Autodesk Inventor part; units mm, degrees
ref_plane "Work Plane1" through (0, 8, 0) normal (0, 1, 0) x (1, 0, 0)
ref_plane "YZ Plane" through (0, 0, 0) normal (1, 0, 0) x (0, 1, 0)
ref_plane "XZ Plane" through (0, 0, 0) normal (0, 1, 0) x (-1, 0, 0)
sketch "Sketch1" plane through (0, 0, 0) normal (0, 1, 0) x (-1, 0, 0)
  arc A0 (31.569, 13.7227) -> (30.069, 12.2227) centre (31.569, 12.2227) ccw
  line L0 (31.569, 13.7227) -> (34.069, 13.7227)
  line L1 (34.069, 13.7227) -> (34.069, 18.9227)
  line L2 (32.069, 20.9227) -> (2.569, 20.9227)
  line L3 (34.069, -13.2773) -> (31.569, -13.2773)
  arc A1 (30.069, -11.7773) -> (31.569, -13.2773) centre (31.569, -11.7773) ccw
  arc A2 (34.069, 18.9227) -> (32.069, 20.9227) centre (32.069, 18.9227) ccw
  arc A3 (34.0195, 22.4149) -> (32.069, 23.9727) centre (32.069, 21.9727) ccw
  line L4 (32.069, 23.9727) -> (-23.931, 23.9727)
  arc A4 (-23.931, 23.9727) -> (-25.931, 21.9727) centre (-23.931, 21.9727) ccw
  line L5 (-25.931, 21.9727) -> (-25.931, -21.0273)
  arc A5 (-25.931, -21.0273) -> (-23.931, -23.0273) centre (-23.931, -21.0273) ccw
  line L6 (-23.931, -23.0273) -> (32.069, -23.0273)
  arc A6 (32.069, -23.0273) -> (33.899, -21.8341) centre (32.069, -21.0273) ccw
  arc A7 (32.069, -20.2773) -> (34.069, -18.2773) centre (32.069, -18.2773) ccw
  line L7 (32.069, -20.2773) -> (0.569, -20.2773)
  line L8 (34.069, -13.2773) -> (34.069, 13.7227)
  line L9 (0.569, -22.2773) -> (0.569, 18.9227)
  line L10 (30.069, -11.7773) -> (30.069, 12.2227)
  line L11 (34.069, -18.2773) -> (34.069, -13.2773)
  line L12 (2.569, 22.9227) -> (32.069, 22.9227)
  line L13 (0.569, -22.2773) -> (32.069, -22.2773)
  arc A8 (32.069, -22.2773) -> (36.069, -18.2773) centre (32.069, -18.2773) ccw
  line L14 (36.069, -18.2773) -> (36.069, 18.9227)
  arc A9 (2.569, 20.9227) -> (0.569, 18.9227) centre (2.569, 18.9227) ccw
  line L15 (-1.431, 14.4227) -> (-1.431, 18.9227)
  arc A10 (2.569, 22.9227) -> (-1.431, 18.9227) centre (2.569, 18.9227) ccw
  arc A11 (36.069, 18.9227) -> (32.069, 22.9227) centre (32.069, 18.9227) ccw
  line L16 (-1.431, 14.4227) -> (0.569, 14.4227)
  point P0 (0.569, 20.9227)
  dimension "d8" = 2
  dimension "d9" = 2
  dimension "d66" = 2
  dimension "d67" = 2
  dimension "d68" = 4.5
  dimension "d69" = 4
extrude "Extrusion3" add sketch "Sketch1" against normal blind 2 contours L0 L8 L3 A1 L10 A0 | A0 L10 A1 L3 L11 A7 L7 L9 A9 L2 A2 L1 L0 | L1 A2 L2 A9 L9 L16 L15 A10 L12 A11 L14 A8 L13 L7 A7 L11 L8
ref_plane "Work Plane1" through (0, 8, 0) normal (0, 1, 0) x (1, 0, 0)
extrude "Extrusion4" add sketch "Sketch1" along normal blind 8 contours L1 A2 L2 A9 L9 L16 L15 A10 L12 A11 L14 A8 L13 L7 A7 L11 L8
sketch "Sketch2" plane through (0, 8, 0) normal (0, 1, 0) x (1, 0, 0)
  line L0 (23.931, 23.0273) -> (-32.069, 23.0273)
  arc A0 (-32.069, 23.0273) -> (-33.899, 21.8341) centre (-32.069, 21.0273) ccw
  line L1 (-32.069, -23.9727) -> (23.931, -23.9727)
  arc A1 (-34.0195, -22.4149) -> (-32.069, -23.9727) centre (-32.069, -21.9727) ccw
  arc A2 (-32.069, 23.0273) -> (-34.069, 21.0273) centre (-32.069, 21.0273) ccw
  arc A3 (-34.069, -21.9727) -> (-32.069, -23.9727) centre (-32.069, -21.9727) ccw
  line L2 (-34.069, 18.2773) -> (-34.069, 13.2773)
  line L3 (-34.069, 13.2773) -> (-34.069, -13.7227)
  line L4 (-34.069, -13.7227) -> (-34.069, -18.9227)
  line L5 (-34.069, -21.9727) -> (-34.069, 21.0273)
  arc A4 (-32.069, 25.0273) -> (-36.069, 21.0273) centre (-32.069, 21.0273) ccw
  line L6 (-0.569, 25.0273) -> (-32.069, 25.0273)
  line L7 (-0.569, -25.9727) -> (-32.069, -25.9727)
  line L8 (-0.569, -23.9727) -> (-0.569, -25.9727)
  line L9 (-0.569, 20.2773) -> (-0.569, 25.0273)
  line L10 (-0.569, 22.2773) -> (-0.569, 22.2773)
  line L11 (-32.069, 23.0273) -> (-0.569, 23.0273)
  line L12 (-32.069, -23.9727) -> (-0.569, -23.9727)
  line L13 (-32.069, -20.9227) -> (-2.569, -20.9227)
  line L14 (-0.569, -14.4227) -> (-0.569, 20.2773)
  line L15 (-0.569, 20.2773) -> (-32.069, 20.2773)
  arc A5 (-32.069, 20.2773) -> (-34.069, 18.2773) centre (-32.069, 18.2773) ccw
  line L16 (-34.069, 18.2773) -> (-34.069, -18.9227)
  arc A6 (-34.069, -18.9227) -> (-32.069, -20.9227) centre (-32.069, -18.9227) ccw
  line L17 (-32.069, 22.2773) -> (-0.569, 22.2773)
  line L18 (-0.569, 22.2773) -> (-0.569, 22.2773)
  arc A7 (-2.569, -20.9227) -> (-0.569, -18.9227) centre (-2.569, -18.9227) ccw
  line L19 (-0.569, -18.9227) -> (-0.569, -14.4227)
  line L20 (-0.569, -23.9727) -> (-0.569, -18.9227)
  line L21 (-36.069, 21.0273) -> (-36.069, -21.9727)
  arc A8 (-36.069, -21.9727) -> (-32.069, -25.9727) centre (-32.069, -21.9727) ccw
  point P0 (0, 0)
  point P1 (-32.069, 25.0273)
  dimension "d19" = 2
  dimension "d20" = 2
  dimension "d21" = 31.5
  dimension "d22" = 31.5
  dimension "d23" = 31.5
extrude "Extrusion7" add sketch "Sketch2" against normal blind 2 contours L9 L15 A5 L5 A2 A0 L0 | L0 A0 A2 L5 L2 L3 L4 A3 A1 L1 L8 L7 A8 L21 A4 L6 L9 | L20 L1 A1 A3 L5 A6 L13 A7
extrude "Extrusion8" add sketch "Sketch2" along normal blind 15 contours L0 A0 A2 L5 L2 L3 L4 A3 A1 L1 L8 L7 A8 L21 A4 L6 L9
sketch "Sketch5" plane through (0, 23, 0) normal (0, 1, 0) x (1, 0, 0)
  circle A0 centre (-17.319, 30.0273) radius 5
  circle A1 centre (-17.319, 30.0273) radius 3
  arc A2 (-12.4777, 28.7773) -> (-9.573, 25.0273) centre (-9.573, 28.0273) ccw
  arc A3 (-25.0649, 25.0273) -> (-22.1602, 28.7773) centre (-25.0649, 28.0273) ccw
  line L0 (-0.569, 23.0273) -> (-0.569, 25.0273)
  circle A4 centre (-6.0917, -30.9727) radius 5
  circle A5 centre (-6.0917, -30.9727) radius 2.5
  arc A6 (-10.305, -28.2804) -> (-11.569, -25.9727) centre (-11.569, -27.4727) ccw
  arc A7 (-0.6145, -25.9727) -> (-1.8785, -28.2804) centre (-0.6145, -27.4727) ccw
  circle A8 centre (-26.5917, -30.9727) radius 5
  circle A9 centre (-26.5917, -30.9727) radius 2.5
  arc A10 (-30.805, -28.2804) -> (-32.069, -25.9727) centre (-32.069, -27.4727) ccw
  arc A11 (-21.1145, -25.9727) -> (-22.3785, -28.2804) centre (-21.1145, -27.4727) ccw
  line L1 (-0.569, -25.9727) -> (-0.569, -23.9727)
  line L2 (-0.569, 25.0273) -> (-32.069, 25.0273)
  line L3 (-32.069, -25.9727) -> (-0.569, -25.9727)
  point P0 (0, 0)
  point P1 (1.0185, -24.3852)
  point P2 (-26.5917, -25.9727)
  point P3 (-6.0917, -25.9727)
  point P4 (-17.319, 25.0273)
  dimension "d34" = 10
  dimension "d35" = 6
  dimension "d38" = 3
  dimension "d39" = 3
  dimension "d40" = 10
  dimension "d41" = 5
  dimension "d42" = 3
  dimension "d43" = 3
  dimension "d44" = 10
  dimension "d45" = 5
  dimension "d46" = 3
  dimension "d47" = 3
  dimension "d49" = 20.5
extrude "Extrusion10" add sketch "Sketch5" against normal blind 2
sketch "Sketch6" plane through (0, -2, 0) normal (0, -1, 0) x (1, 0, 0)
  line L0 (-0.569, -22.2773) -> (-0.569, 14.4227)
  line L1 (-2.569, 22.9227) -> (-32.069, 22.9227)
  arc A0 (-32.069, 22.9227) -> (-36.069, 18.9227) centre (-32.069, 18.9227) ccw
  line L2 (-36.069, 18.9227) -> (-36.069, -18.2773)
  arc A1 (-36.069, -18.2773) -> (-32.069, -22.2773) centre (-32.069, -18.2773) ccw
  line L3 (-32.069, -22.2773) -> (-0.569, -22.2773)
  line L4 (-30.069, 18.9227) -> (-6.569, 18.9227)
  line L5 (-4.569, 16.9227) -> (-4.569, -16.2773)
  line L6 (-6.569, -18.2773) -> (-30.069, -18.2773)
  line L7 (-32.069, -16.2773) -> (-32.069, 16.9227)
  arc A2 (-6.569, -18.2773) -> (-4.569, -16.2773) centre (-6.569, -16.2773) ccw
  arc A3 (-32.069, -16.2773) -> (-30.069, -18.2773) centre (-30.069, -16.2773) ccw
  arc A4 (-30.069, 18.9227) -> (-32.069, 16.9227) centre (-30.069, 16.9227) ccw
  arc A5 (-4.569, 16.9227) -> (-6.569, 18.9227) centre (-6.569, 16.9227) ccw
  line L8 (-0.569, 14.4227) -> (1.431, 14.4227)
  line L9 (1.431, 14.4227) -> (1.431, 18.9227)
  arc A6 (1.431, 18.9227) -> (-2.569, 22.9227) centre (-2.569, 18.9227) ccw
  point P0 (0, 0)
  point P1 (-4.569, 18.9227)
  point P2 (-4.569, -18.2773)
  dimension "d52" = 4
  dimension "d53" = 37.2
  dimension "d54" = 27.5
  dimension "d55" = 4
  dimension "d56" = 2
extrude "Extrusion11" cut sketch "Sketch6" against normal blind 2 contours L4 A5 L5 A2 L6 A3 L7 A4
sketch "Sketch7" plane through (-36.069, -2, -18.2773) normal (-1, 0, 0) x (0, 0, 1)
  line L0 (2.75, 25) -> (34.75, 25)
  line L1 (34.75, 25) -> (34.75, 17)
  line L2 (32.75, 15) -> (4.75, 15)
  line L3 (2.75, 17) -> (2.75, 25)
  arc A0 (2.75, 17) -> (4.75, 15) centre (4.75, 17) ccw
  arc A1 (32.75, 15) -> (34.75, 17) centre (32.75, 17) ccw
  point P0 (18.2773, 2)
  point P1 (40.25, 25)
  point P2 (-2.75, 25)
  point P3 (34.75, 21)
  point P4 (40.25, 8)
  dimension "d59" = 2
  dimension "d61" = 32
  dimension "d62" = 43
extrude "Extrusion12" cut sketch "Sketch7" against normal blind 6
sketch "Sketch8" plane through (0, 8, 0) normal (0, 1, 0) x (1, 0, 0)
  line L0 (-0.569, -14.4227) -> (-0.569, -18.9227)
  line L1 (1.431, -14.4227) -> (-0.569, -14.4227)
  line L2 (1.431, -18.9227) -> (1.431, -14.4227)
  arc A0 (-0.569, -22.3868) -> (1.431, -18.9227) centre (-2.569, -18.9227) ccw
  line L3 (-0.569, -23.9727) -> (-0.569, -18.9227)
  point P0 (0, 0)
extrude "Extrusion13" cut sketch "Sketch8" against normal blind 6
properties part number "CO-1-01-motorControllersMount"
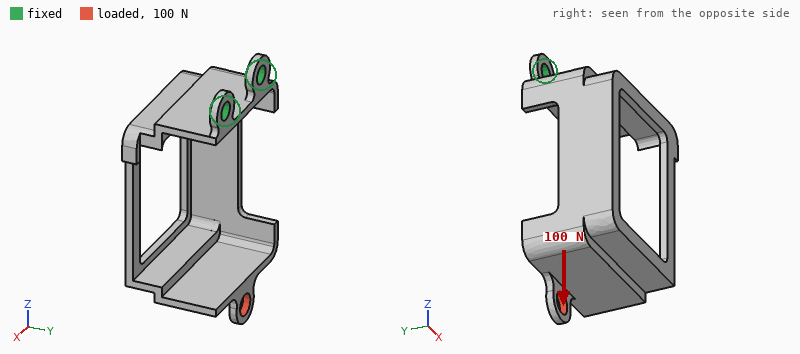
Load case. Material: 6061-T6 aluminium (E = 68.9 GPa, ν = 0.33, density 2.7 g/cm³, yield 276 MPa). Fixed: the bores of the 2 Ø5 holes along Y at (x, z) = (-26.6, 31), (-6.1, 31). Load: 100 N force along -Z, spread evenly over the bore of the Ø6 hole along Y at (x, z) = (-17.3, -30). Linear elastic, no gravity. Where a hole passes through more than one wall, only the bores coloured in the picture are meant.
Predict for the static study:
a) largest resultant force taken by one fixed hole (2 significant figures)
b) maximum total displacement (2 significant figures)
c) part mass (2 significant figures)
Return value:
58 N
1.00 mm
18 g
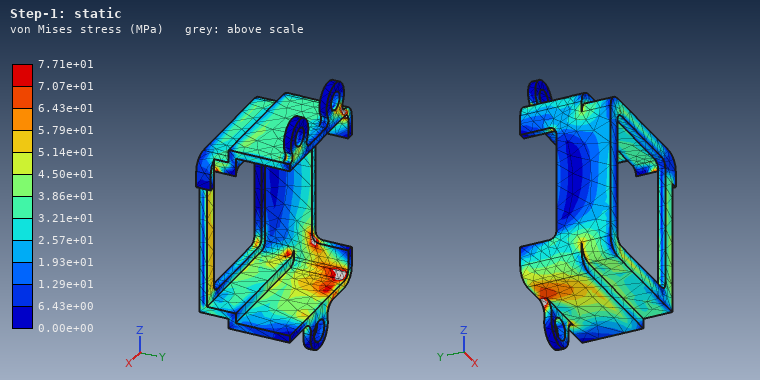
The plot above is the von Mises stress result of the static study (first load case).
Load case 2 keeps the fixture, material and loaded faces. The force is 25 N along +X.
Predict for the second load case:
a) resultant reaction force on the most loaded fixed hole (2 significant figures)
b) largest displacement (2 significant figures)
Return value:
50 N
0.76 mm
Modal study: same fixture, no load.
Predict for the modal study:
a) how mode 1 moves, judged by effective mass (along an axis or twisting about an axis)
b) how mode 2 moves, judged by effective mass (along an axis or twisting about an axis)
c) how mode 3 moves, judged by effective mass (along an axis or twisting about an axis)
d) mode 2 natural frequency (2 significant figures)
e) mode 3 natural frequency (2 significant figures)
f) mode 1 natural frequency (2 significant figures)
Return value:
along Y
along X
along Z
450 Hz
1100 Hz
300 Hz
